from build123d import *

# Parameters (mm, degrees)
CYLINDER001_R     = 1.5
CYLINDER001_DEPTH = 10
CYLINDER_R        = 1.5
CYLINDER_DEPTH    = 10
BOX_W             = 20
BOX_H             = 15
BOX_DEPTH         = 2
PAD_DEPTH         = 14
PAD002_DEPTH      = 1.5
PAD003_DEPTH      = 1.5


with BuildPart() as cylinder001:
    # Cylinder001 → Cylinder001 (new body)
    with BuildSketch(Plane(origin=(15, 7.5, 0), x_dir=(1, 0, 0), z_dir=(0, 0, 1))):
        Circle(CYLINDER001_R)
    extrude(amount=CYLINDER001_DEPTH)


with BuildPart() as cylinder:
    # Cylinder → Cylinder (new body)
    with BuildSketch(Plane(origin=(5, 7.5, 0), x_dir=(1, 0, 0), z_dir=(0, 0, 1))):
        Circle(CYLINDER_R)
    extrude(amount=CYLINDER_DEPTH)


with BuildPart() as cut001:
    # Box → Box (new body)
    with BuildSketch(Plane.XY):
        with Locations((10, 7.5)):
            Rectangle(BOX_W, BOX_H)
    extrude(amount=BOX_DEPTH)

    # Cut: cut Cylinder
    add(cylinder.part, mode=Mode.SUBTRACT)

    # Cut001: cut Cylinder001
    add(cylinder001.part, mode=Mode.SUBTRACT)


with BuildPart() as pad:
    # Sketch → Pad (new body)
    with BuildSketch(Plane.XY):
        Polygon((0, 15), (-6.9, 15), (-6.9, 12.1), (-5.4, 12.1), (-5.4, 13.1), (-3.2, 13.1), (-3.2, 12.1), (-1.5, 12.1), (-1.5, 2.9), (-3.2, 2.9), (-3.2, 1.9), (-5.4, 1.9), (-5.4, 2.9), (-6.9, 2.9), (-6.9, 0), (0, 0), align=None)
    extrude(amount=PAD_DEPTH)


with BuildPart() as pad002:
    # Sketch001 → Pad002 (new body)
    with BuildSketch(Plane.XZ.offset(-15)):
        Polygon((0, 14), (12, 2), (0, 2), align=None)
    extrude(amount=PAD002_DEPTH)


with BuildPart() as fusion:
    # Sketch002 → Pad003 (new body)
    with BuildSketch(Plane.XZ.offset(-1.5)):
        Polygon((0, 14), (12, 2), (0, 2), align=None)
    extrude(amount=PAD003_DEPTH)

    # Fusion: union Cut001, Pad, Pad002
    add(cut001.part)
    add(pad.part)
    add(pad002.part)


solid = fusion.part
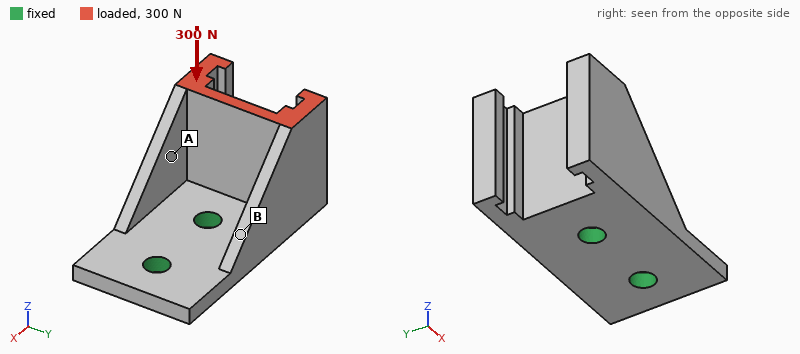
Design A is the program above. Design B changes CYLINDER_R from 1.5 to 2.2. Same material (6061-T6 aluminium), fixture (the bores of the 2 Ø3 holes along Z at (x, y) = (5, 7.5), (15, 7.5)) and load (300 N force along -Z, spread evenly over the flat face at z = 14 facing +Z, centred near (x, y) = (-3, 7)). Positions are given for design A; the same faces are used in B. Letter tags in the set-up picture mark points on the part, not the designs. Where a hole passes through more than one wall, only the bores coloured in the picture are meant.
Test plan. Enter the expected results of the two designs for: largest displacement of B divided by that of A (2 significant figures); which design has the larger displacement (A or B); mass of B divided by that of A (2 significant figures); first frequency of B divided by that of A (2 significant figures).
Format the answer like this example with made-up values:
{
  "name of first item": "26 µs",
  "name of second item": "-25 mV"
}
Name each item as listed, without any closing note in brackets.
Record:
{
  "largest displacement of B divided by that of A": "0.74",
  "which design has the larger displacement": "A",
  "mass of B divided by that of A": "0.99",
  "first frequency of B divided by that of A": "1.2"
}
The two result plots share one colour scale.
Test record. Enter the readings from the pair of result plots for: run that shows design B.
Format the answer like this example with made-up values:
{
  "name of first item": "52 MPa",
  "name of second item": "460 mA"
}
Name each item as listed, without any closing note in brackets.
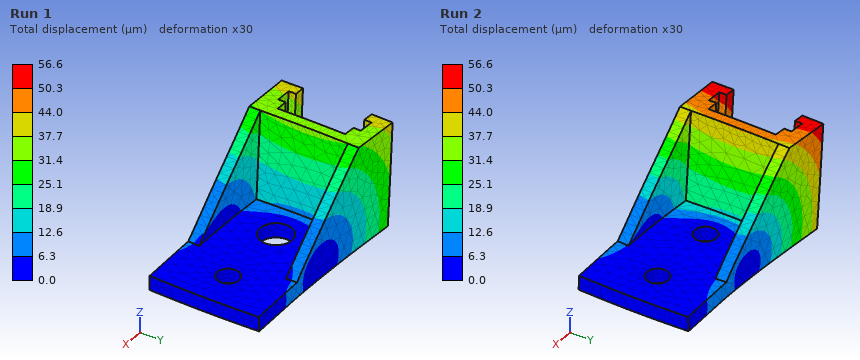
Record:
{
  "run that shows design B": "Run 1"
}
